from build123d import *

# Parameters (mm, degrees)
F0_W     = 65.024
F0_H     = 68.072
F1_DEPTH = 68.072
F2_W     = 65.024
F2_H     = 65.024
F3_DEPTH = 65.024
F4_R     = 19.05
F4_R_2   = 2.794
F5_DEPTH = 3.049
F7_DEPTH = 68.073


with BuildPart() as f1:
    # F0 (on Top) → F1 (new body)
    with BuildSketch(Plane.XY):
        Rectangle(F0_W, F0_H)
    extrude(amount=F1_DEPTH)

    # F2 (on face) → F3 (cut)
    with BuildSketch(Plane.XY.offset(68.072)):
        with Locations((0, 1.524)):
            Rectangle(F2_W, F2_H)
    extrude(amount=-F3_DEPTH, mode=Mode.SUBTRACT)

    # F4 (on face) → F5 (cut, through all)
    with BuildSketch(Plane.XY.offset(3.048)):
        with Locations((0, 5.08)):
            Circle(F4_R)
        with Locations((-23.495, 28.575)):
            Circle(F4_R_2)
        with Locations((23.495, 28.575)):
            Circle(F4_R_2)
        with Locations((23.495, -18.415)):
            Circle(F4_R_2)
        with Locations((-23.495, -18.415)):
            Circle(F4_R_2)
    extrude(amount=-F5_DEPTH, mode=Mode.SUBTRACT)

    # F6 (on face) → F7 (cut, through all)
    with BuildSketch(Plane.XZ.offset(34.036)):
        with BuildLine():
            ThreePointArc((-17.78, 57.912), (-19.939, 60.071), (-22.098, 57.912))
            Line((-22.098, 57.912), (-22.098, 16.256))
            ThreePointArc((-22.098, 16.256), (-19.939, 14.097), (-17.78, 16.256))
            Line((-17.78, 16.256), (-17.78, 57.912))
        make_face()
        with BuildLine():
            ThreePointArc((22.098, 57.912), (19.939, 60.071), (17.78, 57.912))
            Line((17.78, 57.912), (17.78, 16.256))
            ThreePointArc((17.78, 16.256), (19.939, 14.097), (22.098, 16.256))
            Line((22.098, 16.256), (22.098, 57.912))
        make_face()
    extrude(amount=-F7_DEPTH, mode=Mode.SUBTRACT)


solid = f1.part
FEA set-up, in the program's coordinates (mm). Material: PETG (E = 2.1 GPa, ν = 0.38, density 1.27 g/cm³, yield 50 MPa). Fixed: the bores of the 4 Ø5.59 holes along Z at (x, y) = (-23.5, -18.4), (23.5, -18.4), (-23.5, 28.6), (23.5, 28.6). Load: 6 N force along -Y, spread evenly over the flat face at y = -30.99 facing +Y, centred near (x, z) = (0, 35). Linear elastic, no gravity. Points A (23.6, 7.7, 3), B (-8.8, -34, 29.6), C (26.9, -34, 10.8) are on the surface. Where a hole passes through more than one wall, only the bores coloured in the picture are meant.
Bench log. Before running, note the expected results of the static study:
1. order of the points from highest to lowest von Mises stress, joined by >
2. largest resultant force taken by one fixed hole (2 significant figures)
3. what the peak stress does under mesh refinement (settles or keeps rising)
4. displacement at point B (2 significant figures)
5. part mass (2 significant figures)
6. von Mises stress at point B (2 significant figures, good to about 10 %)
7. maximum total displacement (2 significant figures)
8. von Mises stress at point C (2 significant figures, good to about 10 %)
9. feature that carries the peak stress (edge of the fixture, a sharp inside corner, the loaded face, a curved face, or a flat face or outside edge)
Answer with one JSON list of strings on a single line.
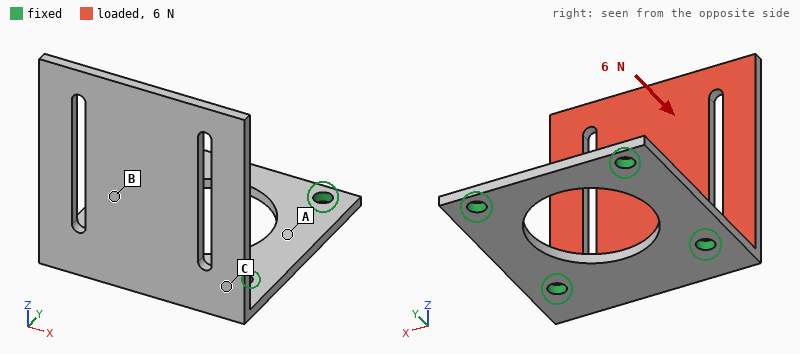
["C > B > A", "3.3 N", "keeps rising", "0.41 mm", "27 g", "0.73 MPa", "1.2 mm", "1.4 MPa", "edge of the fixture"]
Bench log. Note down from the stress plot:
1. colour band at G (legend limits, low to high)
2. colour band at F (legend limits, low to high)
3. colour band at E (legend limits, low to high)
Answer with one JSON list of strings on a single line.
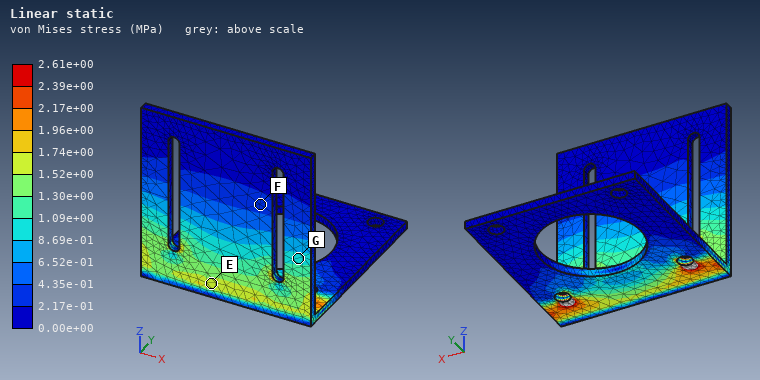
["8.69e-01 to 1.09e+00 MPa", "2.17e-01 to 4.35e-01 MPa", "1.52e+00 to 1.74e+00 MPa"]
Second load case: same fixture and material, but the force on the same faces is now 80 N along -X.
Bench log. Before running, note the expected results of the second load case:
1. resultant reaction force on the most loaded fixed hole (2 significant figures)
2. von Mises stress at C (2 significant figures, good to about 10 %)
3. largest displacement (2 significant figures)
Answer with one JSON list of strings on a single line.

["71 N", "2.9 MPa", "1.2 mm"]
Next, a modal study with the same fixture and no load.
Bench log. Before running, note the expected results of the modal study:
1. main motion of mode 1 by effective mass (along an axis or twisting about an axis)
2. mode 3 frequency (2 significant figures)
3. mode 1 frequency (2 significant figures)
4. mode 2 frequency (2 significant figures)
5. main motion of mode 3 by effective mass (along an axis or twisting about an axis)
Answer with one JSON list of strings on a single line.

["along Y", "510 Hz", "110 Hz", "300 Hz", "along X"]
